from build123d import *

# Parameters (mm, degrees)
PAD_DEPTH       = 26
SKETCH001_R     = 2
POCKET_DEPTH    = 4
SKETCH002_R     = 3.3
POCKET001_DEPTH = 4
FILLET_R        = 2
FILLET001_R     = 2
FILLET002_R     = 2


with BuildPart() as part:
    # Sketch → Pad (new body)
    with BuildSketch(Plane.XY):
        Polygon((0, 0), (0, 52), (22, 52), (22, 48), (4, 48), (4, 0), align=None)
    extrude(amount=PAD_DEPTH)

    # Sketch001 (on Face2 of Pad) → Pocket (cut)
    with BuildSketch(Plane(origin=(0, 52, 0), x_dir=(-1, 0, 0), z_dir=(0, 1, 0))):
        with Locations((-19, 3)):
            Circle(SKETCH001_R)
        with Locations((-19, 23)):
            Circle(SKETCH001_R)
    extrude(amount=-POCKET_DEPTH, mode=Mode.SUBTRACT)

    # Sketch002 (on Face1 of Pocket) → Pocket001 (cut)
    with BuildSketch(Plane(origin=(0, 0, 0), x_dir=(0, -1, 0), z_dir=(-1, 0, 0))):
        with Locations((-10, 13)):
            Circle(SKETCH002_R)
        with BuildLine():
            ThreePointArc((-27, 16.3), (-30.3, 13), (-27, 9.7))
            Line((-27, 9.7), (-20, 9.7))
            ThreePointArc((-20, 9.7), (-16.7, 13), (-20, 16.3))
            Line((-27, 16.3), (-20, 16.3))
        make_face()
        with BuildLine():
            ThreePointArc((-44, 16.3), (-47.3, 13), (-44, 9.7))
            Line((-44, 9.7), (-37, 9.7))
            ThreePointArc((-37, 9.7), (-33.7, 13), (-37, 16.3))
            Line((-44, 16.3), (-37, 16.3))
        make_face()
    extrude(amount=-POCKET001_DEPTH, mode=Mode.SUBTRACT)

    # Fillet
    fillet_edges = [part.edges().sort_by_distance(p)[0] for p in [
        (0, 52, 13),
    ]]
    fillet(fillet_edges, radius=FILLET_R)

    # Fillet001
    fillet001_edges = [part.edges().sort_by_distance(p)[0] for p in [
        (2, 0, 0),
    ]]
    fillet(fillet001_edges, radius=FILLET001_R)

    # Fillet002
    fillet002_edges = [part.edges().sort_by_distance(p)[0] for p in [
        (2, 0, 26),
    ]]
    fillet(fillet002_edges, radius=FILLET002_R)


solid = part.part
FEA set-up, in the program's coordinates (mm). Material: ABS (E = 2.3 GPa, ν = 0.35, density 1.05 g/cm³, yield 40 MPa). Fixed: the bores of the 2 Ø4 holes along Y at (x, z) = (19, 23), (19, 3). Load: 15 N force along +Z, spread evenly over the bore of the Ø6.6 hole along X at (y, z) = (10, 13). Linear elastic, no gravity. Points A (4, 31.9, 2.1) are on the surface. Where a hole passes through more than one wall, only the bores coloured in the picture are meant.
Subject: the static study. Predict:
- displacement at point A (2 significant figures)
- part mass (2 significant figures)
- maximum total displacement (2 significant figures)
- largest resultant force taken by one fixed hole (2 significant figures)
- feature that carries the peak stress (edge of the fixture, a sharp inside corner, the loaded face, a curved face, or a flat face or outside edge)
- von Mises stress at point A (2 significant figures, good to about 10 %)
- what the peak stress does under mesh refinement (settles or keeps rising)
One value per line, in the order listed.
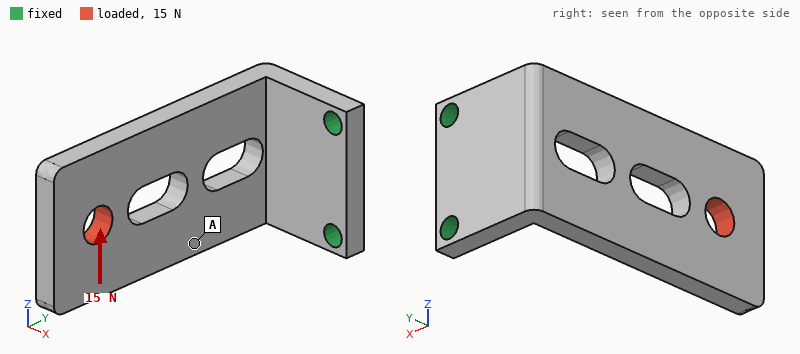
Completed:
0.25 mm
6.7 g
0.61 mm
33 N
edge of the fixture
1.1 MPa
keeps rising
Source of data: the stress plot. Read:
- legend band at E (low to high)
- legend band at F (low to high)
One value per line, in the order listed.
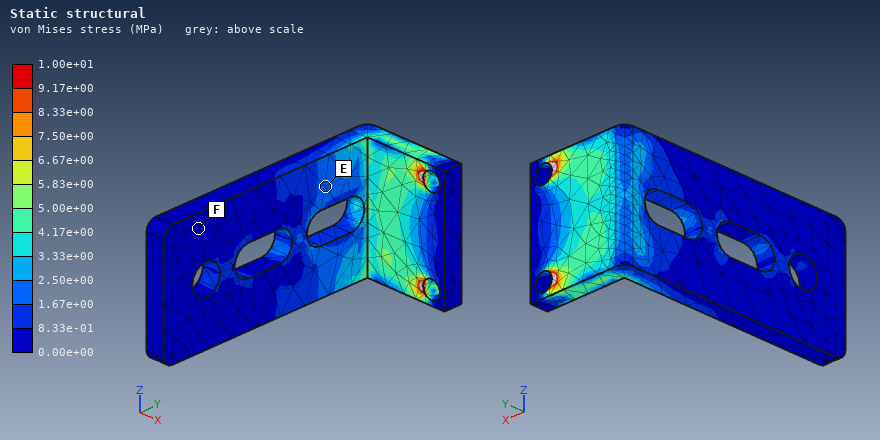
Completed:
1.67e+00 to 2.50e+00 MPa
0.00e+00 to 8.33e-01 MPa
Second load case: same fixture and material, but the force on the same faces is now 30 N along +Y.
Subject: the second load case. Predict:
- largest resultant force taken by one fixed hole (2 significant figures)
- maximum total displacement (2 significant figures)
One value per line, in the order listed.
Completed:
15 N
0.70 mm
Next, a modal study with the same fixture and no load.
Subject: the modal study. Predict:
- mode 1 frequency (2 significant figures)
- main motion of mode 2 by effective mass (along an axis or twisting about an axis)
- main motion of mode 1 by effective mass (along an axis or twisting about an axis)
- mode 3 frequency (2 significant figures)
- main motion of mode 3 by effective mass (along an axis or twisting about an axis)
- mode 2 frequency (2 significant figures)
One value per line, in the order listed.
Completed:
250 Hz
along Z
along X
1200 Hz
along Y
550 Hz
